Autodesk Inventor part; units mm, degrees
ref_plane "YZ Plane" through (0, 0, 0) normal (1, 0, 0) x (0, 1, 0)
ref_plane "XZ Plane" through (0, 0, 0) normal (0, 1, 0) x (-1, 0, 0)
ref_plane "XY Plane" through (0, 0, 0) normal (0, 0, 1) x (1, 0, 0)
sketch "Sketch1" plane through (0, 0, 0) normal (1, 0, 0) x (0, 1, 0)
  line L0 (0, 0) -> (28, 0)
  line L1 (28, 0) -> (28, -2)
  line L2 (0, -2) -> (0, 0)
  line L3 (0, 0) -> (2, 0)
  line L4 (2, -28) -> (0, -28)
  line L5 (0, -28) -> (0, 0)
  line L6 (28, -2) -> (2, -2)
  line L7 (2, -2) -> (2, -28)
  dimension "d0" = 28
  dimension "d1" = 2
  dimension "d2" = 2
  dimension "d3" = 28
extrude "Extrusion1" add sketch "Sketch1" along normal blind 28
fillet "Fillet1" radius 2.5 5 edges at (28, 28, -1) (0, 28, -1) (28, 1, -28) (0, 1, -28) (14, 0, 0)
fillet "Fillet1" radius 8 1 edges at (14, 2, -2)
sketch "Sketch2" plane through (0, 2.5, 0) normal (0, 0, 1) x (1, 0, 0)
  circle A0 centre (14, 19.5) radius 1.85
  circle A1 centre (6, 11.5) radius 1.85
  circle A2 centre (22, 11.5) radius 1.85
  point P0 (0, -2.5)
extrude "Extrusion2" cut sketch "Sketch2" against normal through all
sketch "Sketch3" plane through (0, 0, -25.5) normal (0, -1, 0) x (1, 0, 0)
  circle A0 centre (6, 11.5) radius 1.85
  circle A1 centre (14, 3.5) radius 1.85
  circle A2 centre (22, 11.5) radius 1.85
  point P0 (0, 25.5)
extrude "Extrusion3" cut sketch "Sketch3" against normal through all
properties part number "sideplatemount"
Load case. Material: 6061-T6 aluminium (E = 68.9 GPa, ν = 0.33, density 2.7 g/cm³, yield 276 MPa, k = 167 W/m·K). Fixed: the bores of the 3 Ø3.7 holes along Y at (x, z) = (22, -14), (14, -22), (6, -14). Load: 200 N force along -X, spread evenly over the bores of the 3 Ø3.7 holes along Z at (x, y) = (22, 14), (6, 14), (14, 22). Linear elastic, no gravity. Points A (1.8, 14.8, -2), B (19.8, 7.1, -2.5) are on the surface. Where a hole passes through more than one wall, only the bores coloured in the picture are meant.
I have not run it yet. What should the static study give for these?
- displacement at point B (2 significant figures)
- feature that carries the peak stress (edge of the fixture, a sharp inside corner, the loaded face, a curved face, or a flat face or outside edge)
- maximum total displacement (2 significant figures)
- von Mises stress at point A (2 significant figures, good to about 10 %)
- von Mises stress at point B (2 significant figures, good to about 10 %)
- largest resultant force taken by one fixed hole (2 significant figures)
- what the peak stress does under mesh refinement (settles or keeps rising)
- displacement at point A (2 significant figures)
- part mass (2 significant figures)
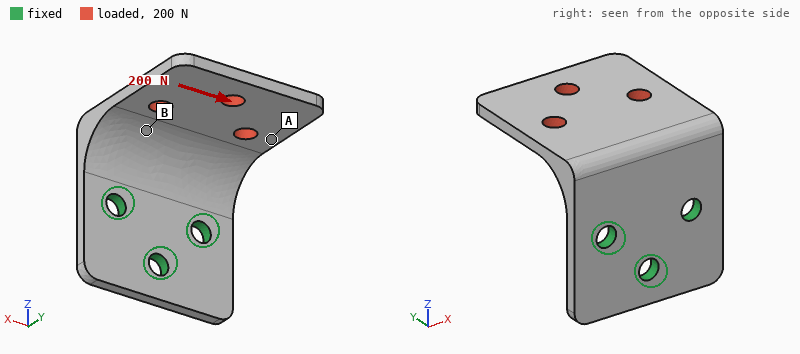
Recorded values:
23 µm
edge of the fixture
87 µm
12 MPa
28 MPa
240 N
keeps rising
55 µm
8.7 g
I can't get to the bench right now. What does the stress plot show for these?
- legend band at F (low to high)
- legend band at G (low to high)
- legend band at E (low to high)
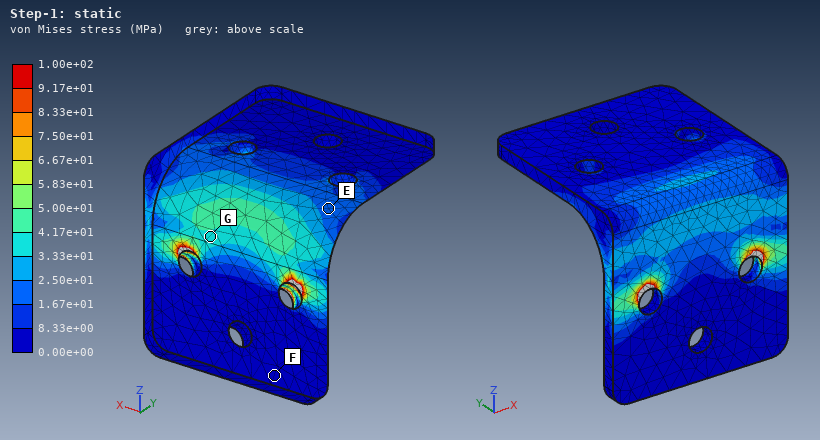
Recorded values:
0.00e+00 to 8.33e+00 MPa
3.33e+01 to 4.17e+01 MPa
1.67e+01 to 2.50e+01 MPa
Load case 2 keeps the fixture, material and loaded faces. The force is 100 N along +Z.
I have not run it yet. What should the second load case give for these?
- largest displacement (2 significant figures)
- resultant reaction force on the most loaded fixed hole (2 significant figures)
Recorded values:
0.30 mm
47 N
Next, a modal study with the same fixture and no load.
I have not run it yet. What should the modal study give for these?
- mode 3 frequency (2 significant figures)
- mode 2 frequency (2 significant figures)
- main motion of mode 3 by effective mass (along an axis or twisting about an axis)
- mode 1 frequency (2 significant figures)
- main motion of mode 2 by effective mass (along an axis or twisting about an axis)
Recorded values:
5900 Hz
4400 Hz
along Y
1800 Hz
along X
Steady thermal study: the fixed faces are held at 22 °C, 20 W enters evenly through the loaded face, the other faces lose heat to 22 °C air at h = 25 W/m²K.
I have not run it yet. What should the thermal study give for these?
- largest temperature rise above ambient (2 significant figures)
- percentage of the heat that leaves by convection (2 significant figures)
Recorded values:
49 K
7.9 %
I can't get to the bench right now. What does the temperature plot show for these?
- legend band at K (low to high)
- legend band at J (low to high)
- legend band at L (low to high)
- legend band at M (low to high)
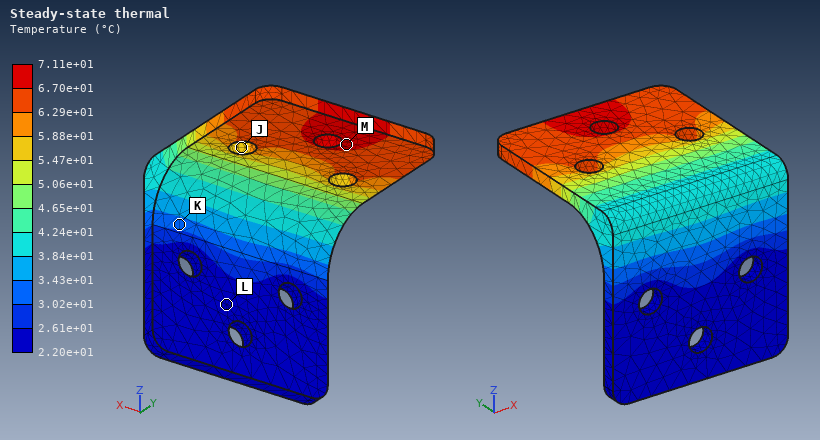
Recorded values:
3.02e+01 to 3.43e+01 °C
5.47e+01 to 5.88e+01 °C
2.20e+01 to 2.61e+01 °C
6.70e+01 to 7.11e+01 °C
